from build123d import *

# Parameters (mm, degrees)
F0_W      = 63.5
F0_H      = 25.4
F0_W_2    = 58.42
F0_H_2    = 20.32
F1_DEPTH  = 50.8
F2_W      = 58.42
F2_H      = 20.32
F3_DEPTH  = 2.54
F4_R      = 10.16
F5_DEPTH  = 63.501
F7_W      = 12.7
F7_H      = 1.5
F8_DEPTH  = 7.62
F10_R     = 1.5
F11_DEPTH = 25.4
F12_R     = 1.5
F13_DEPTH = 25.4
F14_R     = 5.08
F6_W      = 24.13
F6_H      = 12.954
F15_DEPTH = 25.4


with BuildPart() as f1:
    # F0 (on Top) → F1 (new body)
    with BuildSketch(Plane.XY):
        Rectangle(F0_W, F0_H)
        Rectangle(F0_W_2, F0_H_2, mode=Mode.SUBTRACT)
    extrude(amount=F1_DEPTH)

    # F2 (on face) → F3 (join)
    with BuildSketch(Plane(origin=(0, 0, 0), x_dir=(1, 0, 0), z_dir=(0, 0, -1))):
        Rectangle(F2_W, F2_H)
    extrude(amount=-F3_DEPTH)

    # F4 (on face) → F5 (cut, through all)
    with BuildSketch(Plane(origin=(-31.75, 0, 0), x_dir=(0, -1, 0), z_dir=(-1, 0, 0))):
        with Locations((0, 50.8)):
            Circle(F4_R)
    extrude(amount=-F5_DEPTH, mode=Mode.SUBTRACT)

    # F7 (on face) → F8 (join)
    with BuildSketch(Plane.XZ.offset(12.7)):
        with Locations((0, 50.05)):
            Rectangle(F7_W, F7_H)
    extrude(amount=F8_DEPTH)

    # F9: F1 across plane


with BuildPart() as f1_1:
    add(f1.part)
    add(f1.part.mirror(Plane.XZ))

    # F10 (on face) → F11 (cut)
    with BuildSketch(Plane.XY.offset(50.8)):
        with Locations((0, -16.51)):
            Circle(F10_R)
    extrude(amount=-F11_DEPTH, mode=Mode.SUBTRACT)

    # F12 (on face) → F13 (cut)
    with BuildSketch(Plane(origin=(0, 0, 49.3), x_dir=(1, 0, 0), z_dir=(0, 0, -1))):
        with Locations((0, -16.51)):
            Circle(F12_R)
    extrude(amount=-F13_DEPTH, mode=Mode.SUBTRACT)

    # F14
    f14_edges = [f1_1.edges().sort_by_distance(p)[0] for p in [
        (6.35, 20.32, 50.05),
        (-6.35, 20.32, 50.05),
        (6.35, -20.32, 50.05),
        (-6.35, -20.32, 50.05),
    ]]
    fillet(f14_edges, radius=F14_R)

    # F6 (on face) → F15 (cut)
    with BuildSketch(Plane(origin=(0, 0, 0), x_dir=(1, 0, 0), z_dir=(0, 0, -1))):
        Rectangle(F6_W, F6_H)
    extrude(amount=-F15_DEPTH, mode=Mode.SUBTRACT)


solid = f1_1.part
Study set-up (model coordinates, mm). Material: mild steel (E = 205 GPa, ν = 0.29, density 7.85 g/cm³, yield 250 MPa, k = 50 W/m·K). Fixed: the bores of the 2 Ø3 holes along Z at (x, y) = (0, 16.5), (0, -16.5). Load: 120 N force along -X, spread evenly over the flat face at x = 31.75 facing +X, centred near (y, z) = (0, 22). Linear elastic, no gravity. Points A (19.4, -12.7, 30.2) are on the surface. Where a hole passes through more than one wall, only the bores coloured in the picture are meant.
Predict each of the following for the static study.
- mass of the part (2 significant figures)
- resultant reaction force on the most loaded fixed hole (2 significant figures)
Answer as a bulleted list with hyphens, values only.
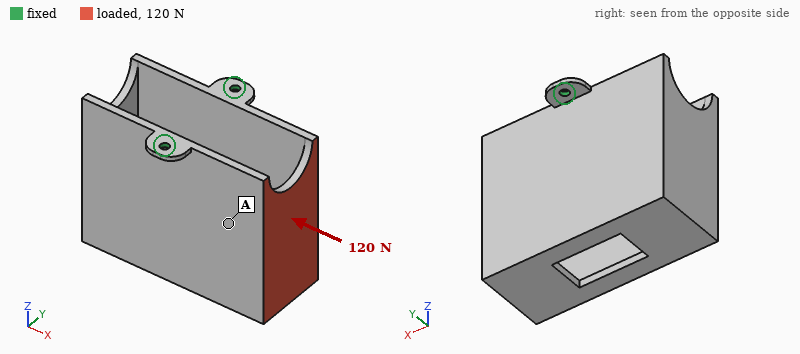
- 180 g
- 60 N
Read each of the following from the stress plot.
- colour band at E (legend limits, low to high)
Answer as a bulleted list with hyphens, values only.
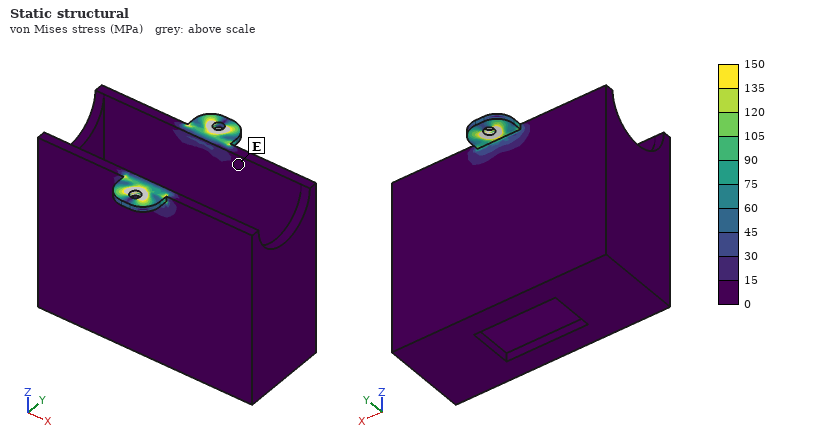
- 0 to 15 MPa
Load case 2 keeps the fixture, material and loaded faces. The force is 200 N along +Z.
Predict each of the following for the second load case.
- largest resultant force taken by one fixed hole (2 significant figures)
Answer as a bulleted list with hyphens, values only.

- 100 N
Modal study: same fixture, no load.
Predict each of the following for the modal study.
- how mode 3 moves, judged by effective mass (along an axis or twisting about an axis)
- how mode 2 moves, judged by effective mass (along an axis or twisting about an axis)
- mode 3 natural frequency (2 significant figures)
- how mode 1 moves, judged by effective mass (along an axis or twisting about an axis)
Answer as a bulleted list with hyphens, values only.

- twisting about Z
- along Y
- 1600 Hz
- along X
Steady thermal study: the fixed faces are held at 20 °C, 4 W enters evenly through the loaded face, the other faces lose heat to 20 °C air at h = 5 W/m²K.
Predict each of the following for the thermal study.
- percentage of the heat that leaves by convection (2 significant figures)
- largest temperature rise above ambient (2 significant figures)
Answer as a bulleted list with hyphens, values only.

- 32 %
- 22 K
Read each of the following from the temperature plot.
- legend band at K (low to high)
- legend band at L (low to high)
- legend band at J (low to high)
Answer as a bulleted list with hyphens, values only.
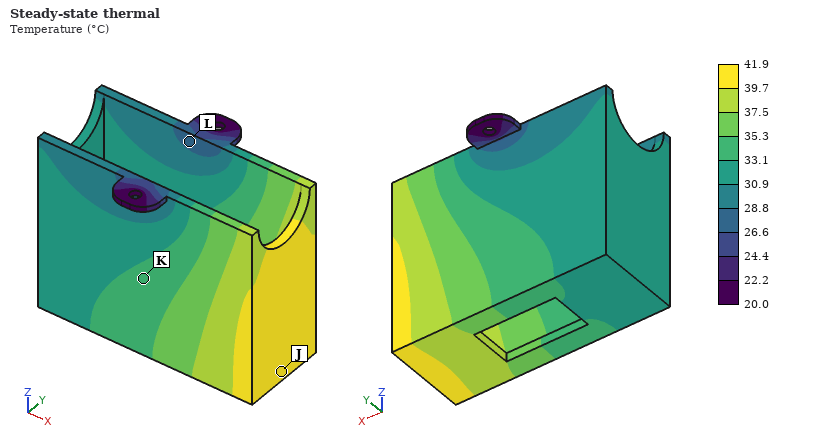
- 33.1 to 35.3 °C
- 26.6 to 28.8 °C
- 39.7 to 41.9 °C
